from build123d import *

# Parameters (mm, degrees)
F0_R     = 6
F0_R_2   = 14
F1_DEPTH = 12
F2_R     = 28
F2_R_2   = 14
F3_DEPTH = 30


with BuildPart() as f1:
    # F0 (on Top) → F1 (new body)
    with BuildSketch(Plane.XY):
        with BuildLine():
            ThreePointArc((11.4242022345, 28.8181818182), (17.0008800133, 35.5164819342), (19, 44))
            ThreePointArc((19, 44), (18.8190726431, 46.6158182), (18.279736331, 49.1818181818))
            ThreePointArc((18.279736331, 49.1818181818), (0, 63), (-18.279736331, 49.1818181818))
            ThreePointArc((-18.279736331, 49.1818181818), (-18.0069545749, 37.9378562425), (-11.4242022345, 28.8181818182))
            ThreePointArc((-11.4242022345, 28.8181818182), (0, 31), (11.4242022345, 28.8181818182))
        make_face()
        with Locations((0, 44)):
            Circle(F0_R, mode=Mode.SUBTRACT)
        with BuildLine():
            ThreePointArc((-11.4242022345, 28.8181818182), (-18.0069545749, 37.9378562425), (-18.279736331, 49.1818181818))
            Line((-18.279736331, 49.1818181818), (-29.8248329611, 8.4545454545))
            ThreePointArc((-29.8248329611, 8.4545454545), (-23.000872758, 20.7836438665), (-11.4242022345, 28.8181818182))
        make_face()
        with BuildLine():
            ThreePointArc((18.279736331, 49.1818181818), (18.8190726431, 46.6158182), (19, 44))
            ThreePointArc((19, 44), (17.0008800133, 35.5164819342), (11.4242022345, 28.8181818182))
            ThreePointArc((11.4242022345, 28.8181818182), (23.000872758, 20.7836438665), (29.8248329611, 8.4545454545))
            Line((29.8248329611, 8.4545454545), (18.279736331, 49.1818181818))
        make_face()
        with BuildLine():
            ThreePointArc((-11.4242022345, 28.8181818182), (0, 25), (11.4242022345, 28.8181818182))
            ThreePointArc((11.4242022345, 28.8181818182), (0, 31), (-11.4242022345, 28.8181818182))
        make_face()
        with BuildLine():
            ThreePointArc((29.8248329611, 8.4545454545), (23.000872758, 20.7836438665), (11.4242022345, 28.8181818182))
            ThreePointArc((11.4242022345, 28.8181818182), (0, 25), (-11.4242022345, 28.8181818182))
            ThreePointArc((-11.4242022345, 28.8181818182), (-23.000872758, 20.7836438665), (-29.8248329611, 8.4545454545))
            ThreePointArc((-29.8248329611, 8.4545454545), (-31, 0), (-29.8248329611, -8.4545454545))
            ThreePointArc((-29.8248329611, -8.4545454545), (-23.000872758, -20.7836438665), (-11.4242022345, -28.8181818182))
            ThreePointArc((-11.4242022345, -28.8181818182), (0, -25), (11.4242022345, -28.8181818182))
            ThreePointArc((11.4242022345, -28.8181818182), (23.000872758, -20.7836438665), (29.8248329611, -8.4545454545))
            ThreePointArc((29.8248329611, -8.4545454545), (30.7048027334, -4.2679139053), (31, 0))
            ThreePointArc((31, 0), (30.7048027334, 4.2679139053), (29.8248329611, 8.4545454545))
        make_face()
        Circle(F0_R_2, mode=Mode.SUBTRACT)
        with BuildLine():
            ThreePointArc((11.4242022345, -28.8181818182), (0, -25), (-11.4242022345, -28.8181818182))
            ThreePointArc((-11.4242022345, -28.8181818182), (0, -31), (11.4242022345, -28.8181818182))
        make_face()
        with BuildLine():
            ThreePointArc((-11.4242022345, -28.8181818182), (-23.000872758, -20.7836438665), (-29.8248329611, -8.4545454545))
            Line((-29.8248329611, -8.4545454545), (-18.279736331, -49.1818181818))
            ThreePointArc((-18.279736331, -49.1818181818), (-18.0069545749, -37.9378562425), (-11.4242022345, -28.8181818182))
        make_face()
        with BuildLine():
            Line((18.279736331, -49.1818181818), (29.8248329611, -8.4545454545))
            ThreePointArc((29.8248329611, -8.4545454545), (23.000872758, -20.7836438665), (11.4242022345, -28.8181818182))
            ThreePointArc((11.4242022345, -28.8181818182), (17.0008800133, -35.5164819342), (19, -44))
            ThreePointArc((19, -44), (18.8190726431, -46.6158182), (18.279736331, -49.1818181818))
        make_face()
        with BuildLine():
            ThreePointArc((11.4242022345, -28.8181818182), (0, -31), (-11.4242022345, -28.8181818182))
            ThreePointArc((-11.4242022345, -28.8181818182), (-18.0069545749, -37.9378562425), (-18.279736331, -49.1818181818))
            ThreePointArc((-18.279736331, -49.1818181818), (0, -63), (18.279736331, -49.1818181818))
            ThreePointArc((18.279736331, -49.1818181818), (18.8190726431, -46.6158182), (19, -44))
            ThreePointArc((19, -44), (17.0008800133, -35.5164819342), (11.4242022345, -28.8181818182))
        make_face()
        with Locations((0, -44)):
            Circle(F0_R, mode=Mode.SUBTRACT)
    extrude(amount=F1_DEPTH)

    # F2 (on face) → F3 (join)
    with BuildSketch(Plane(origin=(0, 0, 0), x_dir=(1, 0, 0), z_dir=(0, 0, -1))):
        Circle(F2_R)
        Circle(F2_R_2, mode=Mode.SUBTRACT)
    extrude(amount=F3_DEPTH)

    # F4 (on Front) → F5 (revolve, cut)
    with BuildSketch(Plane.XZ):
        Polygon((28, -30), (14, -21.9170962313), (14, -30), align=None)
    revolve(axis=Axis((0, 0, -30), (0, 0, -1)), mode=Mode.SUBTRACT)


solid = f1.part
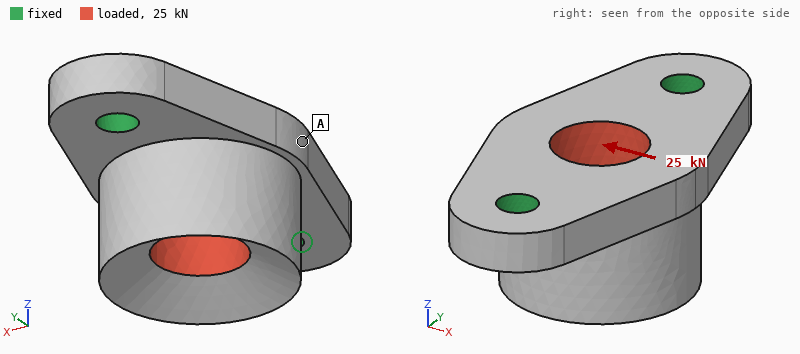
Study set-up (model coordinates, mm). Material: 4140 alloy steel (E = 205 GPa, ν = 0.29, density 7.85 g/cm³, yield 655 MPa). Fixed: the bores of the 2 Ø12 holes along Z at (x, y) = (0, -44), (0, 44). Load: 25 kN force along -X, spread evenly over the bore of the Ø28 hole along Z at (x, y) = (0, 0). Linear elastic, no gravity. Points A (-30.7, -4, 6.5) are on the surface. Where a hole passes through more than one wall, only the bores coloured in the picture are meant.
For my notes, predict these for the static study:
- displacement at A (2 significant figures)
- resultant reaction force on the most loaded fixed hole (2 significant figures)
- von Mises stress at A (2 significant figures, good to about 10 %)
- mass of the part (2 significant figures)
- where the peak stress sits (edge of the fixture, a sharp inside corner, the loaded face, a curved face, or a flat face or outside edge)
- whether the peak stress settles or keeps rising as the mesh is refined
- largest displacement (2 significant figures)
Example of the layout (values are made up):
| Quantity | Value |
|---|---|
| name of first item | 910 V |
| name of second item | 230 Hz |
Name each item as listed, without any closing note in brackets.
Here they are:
| Quantity | Value |
|---|---|
| displacement at A | 42 µm |
| resultant reaction force on the most loaded fixed hole | 13 kN |
| von Mises stress at A | 27 MPa |
| mass of the part | 840 g |
| where the peak stress sits | edge of the fixture |
| whether the peak stress settles or keeps rising as the mesh is refined | keeps rising |
| largest displacement | 71 µm |
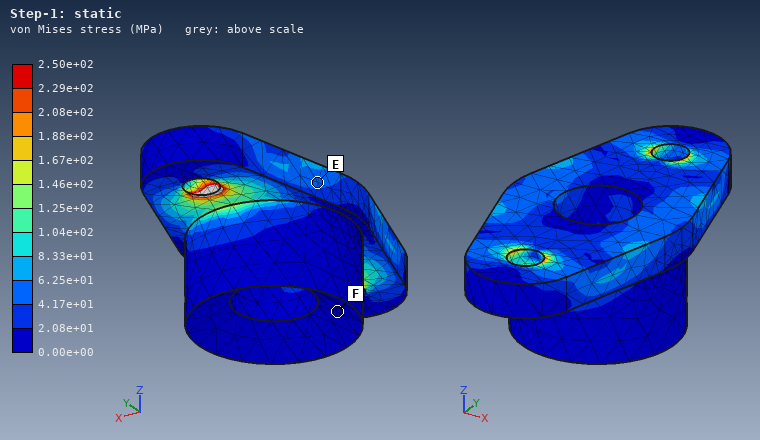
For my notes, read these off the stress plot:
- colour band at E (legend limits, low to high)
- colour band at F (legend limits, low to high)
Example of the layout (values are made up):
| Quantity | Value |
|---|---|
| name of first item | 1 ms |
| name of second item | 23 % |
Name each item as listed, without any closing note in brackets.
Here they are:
| Quantity | Value |
|---|---|
| colour band at E | 4.17e+01 to 6.25e+01 MPa |
| colour band at F | 0.00e+00 to 2.08e+01 MPa |
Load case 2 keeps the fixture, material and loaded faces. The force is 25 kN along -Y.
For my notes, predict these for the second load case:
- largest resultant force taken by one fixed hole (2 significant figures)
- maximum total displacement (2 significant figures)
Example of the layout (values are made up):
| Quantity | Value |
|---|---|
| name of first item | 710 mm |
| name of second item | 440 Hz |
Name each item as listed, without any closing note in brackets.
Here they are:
| Quantity | Value |
|---|---|
| largest resultant force taken by one fixed hole | 13 kN |
| maximum total displacement | 11 µm |
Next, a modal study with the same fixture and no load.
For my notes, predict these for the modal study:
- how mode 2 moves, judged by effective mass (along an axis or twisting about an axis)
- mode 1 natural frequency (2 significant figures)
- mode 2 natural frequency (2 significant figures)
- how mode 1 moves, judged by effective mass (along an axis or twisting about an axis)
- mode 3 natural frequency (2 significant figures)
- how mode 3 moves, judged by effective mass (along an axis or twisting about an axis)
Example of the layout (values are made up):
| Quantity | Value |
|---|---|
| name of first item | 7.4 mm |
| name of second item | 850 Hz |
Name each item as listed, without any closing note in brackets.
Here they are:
| Quantity | Value |
|---|---|
| how mode 2 moves, judged by effective mass | along Z |
| mode 1 natural frequency | 3800 Hz |
| mode 2 natural frequency | 6800 Hz |
| how mode 1 moves, judged by effective mass | along X |
| mode 3 natural frequency | 10 kHz |
| how mode 3 moves, judged by effective mass | along Y |
